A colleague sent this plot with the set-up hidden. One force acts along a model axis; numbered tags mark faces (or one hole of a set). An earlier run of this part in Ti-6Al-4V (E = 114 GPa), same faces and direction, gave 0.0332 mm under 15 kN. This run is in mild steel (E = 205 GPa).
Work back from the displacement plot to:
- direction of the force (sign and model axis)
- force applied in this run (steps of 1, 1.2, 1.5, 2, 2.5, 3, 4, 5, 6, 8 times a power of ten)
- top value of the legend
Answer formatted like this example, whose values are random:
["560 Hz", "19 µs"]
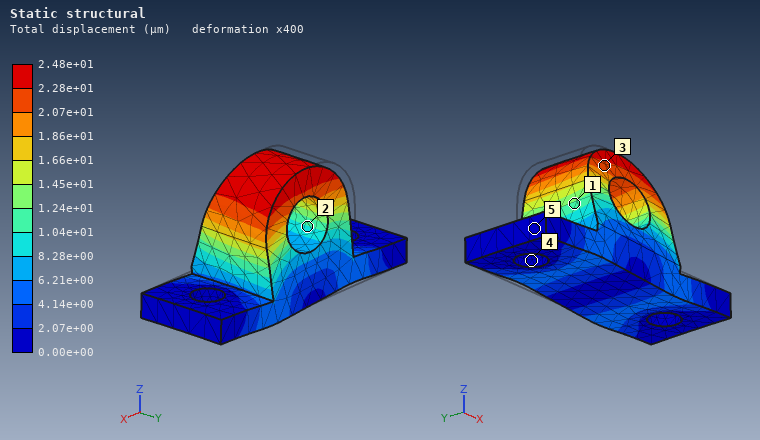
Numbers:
["+X", "20 kN", "2.48e+01 µm"]
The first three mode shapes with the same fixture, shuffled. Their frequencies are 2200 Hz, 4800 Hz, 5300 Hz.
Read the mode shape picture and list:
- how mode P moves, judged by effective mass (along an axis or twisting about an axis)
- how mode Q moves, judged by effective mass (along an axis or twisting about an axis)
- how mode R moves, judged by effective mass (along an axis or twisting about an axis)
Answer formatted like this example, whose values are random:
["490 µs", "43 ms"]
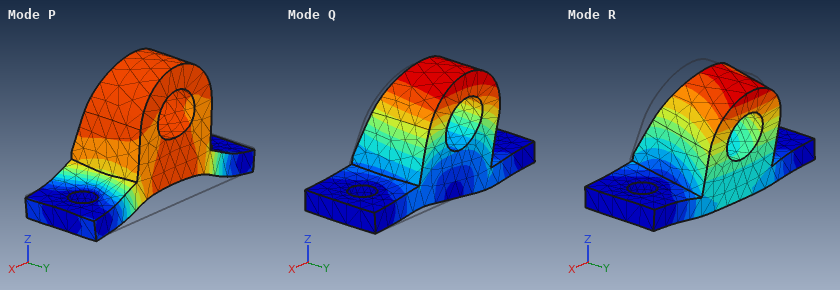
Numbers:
["along Z", "along X", "along Y"]
